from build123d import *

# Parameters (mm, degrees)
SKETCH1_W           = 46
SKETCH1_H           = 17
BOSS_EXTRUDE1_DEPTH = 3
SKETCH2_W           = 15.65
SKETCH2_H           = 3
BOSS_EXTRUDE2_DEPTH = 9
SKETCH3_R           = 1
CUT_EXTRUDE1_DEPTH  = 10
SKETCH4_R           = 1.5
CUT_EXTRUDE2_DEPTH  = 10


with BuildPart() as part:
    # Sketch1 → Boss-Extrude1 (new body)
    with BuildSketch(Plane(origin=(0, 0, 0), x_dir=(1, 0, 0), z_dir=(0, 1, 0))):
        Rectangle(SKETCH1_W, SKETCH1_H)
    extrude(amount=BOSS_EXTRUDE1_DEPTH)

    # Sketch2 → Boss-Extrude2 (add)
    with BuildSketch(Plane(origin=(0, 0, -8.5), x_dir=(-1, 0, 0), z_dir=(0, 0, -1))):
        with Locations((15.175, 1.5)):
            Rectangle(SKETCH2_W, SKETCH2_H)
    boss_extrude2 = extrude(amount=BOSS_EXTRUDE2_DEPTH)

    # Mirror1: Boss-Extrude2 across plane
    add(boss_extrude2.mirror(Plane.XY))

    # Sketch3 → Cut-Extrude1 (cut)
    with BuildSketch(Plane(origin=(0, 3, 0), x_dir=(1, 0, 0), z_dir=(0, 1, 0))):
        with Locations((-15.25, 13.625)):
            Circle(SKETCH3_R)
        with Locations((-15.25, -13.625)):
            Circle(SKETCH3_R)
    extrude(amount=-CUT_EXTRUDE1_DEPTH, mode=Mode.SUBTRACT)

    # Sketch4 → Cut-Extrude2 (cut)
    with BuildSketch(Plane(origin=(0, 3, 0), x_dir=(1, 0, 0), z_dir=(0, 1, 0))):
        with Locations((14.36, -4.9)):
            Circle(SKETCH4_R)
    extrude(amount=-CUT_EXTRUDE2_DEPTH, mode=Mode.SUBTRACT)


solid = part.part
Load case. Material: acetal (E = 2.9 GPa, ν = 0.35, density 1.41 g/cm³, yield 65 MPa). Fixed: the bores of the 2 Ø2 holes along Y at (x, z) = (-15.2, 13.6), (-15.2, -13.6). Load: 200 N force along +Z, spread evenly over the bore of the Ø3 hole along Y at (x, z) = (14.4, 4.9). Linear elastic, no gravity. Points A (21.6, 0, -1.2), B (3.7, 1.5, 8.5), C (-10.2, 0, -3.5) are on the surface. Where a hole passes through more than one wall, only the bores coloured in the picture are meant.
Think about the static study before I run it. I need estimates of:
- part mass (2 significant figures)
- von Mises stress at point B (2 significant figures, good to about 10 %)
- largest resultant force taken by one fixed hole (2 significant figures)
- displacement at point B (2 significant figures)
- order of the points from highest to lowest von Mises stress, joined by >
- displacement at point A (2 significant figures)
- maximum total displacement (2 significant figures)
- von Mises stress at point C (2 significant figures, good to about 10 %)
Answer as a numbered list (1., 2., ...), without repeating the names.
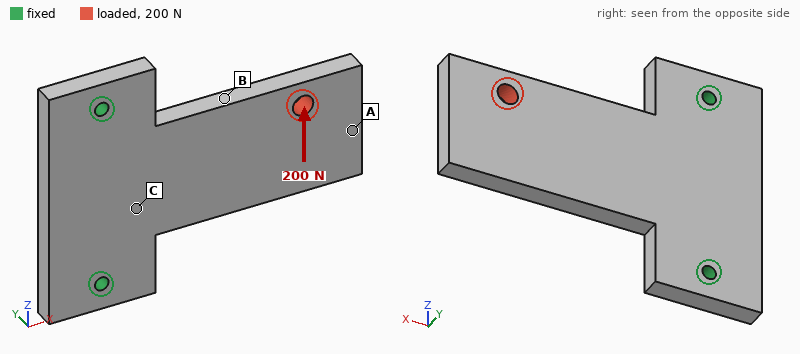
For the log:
1. 4.4 g
2. 15 MPa
3. 240 N
4. 0.27 mm
5. B > C > A
6. 0.62 mm
7. 0.68 mm
8. 6.8 MPa
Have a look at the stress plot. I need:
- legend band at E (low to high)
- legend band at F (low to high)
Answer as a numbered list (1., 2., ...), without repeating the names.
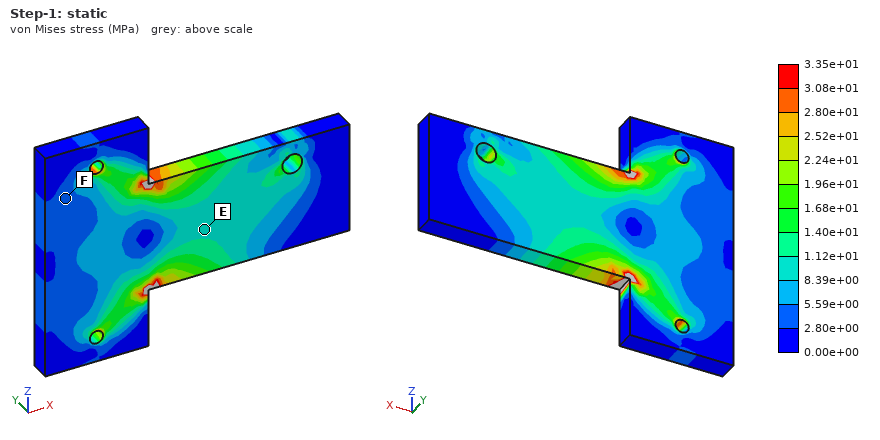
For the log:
1. 8.39e+00 to 1.12e+01 MPa
2. 2.80e+00 to 5.59e+00 MPa
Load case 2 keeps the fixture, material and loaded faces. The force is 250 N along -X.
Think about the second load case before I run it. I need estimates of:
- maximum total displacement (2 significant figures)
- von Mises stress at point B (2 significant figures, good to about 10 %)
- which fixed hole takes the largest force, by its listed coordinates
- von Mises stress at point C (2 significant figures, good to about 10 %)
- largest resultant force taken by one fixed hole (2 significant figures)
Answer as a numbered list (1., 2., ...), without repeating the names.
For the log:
1. 0.26 mm
2. 13 MPa
3. (-15.2, 13.6)
4. 4.0 MPa
5. 170 N
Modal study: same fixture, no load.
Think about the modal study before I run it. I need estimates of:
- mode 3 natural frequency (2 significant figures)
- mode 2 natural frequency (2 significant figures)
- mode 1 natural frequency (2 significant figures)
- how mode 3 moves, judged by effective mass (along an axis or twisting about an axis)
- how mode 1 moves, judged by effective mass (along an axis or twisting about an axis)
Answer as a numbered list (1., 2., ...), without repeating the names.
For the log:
1. 2600 Hz
2. 2200 Hz
3. 460 Hz
4. along Y
5. along Y
